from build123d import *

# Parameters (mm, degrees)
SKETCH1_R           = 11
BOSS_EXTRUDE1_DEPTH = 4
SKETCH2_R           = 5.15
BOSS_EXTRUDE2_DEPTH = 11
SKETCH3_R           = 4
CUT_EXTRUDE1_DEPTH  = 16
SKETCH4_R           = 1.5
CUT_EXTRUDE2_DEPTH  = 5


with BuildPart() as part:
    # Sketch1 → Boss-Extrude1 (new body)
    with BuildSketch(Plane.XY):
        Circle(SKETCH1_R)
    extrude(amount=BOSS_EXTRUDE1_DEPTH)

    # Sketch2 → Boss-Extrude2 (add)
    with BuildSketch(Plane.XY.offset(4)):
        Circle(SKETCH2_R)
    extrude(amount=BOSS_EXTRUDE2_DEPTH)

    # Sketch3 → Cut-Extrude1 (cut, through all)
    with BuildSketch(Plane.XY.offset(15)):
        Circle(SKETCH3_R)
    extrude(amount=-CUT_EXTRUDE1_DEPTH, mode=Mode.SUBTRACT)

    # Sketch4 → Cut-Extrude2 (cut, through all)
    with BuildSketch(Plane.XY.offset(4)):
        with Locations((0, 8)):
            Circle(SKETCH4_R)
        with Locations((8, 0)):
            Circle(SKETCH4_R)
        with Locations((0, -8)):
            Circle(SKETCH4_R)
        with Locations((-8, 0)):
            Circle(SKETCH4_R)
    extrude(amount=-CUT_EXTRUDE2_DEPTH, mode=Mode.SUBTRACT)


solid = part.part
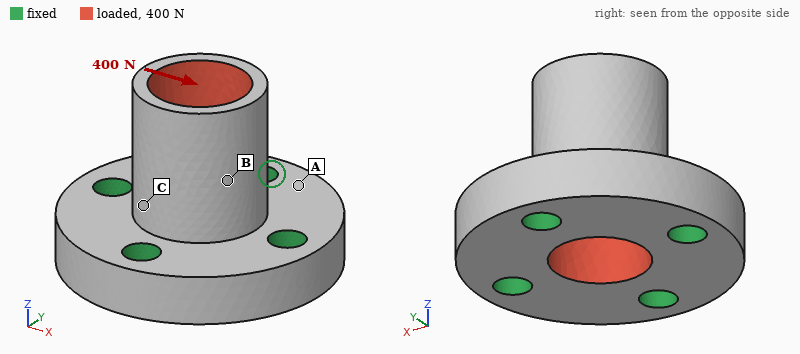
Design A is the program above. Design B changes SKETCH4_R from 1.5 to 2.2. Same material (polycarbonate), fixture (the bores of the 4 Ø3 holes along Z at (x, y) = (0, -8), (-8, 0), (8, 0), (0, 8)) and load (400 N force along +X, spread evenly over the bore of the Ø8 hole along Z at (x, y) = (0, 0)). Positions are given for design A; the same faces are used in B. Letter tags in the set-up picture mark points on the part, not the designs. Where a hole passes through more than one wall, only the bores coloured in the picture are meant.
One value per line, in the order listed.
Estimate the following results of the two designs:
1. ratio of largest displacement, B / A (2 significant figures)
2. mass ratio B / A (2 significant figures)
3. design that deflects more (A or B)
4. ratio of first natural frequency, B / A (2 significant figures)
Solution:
0.92
0.92
A
1.0
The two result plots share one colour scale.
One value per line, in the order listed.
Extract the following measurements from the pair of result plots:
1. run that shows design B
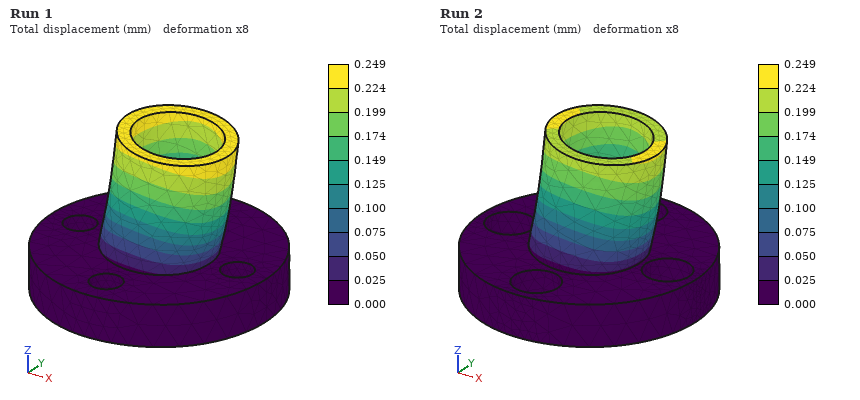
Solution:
Run 2
